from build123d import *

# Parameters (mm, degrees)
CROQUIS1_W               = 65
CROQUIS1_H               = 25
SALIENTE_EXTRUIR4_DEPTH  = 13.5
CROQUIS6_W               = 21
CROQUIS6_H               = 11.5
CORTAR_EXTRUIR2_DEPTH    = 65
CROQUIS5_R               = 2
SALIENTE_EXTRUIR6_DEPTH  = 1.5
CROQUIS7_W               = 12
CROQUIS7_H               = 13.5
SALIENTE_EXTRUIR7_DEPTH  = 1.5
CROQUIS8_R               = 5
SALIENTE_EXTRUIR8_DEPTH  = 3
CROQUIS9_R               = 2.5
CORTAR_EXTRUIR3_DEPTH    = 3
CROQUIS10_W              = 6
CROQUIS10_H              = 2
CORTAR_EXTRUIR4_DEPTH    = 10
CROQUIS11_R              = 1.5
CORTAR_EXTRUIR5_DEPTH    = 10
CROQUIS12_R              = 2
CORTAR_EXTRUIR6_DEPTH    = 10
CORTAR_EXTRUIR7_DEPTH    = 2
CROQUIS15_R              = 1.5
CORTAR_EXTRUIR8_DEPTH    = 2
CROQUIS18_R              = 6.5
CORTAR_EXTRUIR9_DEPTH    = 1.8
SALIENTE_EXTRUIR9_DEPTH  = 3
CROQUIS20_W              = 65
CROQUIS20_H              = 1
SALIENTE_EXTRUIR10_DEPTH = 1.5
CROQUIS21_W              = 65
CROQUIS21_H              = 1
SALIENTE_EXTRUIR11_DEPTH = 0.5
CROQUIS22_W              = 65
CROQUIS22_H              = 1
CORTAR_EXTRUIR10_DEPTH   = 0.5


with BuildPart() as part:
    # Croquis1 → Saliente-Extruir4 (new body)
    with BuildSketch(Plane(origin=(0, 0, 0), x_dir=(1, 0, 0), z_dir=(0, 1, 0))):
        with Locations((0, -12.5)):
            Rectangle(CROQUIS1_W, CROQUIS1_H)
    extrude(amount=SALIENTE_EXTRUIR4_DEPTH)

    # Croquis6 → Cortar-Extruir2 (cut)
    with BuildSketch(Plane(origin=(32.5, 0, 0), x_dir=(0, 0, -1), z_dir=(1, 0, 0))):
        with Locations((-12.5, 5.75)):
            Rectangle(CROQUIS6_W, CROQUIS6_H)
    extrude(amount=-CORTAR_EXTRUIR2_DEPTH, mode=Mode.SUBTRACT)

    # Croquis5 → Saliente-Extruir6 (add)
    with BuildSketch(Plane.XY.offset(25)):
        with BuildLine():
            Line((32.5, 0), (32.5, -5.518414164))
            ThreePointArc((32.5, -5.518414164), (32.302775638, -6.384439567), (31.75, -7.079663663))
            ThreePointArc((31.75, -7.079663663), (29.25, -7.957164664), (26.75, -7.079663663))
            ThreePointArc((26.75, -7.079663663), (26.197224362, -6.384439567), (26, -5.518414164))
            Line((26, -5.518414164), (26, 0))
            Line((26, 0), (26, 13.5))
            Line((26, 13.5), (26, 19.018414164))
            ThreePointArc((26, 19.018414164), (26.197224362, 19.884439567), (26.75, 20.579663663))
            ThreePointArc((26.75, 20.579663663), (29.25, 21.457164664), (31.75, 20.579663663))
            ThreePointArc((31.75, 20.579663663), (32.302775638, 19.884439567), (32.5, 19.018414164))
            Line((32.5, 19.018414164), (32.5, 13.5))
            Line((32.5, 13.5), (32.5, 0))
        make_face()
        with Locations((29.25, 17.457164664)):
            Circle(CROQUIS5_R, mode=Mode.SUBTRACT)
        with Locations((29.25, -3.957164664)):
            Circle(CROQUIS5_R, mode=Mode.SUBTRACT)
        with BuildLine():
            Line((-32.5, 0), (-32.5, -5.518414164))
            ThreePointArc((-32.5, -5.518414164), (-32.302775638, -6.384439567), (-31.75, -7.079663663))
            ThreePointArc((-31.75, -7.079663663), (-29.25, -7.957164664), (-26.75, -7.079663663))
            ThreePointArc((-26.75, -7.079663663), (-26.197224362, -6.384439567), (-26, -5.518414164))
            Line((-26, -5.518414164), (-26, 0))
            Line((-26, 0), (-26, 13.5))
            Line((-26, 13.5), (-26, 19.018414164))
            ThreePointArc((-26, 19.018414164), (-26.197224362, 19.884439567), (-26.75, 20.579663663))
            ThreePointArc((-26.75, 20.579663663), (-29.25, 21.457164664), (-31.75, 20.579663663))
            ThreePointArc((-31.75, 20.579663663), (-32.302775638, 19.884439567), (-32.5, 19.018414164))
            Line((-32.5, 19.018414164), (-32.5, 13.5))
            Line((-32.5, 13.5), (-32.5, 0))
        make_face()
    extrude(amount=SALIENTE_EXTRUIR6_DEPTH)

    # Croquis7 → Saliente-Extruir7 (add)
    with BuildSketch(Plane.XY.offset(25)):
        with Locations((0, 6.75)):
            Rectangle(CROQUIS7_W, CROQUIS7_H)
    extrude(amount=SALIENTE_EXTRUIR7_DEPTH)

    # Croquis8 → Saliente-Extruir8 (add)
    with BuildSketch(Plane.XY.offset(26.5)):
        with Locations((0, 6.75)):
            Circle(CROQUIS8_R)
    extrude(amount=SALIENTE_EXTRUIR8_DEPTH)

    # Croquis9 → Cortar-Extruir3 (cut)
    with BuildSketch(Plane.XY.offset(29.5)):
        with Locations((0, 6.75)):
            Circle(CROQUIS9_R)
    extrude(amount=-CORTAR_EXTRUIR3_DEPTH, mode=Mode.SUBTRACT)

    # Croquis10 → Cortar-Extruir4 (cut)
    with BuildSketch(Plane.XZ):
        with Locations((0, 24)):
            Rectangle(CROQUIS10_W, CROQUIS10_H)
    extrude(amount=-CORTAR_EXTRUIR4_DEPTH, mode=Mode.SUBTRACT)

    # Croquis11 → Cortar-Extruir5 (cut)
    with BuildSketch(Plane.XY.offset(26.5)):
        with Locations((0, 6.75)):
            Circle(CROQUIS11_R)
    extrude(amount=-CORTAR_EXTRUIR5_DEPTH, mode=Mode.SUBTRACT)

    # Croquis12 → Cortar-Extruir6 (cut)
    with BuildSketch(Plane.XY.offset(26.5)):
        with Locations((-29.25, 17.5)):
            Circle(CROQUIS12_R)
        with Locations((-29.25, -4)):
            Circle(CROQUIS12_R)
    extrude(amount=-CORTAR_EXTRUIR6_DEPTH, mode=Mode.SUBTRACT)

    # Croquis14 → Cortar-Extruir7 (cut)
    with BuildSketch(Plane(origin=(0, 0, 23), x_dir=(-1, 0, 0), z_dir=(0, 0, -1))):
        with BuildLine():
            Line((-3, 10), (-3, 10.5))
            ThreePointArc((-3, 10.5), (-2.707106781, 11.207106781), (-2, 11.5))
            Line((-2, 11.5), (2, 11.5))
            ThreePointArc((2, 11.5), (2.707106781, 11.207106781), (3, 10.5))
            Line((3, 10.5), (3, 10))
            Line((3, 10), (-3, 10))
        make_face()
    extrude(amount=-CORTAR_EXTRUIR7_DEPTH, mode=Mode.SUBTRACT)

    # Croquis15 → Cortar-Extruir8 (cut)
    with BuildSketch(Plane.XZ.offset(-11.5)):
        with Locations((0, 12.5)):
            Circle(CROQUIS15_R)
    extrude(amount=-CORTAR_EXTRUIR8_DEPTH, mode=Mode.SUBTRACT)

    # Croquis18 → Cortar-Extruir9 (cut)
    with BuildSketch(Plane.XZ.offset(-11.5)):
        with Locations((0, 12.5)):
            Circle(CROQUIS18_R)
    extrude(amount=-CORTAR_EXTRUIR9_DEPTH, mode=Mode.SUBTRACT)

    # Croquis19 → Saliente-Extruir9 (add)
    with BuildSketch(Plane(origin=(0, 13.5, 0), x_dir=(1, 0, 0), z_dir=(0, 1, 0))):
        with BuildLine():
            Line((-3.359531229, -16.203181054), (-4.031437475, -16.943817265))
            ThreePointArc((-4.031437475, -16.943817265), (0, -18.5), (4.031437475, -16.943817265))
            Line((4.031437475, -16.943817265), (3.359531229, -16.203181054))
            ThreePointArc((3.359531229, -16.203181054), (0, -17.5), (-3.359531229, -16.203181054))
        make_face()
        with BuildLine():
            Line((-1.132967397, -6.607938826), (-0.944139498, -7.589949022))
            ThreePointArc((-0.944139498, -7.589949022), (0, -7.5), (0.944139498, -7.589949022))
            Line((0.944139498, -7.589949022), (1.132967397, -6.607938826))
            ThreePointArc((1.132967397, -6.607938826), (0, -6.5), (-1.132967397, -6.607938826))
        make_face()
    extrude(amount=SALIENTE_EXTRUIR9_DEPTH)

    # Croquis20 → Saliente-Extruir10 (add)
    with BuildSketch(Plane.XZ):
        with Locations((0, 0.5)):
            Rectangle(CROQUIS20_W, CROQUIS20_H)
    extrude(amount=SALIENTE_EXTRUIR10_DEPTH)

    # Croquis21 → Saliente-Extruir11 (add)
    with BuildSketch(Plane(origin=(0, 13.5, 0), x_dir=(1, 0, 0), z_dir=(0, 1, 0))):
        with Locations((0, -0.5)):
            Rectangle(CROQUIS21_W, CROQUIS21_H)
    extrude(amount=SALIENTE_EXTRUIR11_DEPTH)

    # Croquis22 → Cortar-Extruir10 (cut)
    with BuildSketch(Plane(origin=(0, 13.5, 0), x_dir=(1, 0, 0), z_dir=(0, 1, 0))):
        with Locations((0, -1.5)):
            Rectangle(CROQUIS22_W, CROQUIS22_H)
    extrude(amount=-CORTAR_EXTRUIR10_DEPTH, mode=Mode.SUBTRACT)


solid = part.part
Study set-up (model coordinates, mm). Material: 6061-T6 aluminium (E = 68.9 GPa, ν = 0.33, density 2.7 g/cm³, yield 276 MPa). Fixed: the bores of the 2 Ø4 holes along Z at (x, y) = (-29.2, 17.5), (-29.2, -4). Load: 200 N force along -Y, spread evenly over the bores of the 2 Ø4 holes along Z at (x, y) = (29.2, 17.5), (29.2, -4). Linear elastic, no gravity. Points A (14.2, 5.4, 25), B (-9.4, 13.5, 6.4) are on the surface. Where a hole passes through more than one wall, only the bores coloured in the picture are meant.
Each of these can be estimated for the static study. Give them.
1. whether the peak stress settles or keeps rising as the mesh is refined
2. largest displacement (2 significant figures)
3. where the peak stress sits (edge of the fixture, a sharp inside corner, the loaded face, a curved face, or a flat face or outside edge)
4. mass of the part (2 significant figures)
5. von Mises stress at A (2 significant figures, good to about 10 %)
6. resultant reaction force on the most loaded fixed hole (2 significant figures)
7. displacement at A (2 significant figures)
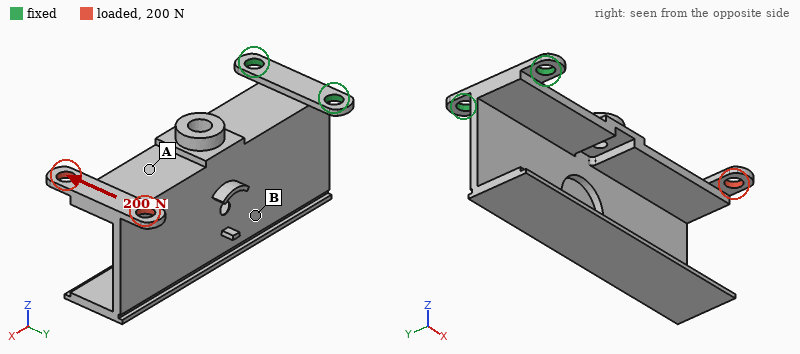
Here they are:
keeps rising
0.59 mm
a sharp inside corner
19 g
46 MPa
680 N
0.33 mm
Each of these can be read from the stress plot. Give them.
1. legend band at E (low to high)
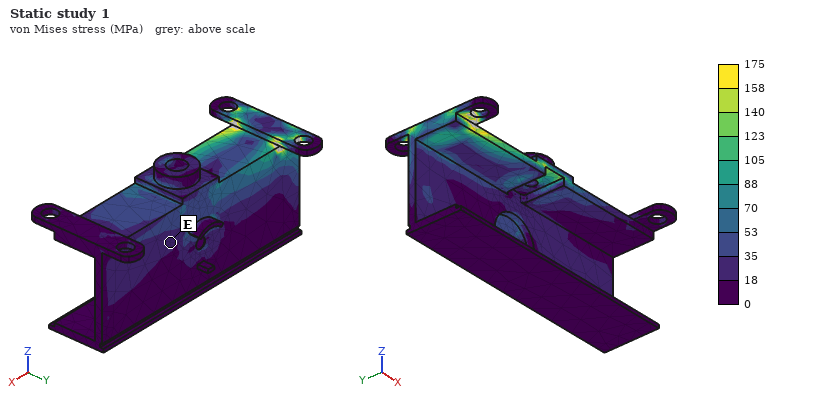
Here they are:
18 to 35 MPa
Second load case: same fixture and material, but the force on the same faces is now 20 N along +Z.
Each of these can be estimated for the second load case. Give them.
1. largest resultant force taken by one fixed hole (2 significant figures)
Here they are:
25 N
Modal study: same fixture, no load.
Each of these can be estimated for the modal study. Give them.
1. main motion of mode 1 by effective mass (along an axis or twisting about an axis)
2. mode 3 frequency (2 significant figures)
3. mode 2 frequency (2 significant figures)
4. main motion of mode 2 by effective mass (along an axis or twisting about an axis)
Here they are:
along Z
1600 Hz
720 Hz
along Y
